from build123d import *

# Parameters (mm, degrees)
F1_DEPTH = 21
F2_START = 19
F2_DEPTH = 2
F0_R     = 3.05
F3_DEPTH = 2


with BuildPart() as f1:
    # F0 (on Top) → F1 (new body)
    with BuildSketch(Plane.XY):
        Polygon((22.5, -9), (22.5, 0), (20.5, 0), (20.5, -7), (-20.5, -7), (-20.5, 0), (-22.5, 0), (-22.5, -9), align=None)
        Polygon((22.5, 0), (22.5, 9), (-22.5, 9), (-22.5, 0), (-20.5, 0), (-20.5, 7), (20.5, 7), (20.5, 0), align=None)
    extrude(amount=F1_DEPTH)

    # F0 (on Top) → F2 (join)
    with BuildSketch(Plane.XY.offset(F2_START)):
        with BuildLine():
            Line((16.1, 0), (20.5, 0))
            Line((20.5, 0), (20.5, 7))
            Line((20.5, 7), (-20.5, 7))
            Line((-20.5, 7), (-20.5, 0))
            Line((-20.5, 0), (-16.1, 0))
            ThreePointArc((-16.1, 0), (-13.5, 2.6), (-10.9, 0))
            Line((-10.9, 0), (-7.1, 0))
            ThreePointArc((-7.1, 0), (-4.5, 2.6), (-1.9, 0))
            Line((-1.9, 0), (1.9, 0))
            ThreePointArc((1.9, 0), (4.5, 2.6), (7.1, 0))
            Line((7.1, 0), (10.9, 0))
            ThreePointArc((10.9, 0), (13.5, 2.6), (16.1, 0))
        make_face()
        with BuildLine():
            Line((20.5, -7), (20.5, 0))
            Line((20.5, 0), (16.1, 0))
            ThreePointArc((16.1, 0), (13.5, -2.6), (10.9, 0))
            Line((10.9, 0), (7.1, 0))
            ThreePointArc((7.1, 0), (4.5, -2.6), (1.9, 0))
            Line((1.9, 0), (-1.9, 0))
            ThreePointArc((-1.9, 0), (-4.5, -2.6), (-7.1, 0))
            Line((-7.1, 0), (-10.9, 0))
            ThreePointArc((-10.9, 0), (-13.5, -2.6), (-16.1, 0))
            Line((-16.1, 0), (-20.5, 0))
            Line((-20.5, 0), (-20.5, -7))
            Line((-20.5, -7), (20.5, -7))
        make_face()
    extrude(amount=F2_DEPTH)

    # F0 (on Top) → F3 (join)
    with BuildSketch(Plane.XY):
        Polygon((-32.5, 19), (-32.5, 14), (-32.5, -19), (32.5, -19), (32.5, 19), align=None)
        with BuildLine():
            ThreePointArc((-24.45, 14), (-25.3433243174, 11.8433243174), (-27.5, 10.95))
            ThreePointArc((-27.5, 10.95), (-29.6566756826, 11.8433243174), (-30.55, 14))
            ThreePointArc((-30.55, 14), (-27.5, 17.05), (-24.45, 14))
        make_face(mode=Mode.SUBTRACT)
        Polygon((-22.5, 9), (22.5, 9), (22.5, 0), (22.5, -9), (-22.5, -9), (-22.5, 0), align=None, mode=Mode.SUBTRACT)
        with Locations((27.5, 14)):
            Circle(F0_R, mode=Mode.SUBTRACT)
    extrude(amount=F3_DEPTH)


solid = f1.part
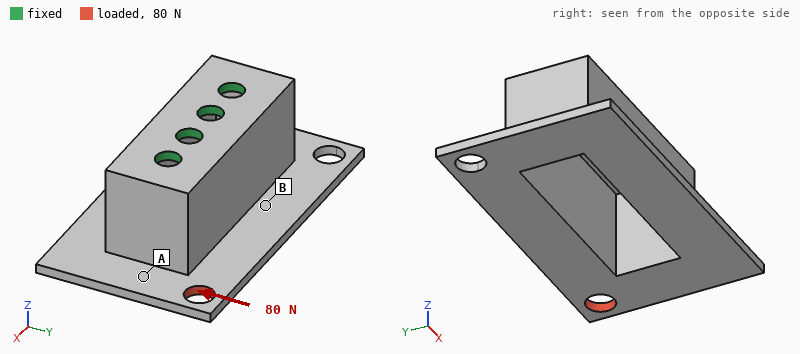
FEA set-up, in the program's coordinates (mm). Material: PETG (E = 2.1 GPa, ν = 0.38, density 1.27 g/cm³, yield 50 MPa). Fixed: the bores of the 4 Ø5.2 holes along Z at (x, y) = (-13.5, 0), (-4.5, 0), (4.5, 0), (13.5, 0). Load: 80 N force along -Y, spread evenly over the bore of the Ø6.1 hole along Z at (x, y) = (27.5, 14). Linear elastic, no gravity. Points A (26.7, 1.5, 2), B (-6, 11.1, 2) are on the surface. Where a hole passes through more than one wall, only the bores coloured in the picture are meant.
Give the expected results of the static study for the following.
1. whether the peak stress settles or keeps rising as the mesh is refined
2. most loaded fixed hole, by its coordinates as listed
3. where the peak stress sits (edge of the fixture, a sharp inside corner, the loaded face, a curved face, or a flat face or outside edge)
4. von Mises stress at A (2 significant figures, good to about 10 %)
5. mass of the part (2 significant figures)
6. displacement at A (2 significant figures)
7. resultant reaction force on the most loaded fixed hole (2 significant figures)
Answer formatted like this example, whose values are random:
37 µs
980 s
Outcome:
keeps rising
(13.5, 0)
edge of the fixture
4.2 MPa
12 g
0.53 mm
120 N
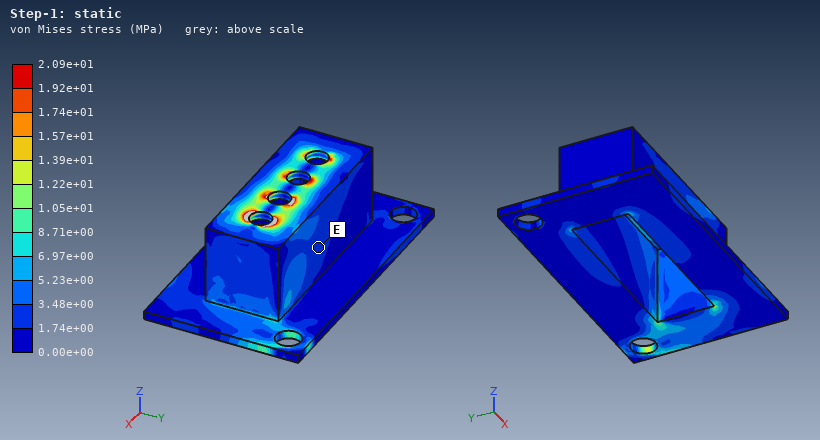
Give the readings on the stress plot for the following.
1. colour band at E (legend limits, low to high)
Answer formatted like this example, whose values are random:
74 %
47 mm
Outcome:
1.74e+00 to 3.48e+00 MPa
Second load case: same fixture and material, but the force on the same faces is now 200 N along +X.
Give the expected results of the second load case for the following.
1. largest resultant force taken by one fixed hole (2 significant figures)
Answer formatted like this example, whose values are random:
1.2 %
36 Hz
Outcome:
140 N
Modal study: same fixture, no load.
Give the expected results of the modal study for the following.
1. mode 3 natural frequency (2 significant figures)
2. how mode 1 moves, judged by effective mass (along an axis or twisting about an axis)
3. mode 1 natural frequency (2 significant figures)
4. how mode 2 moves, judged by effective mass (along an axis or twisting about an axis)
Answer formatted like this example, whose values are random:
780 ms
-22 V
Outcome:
1600 Hz
along Y
790 Hz
along X
